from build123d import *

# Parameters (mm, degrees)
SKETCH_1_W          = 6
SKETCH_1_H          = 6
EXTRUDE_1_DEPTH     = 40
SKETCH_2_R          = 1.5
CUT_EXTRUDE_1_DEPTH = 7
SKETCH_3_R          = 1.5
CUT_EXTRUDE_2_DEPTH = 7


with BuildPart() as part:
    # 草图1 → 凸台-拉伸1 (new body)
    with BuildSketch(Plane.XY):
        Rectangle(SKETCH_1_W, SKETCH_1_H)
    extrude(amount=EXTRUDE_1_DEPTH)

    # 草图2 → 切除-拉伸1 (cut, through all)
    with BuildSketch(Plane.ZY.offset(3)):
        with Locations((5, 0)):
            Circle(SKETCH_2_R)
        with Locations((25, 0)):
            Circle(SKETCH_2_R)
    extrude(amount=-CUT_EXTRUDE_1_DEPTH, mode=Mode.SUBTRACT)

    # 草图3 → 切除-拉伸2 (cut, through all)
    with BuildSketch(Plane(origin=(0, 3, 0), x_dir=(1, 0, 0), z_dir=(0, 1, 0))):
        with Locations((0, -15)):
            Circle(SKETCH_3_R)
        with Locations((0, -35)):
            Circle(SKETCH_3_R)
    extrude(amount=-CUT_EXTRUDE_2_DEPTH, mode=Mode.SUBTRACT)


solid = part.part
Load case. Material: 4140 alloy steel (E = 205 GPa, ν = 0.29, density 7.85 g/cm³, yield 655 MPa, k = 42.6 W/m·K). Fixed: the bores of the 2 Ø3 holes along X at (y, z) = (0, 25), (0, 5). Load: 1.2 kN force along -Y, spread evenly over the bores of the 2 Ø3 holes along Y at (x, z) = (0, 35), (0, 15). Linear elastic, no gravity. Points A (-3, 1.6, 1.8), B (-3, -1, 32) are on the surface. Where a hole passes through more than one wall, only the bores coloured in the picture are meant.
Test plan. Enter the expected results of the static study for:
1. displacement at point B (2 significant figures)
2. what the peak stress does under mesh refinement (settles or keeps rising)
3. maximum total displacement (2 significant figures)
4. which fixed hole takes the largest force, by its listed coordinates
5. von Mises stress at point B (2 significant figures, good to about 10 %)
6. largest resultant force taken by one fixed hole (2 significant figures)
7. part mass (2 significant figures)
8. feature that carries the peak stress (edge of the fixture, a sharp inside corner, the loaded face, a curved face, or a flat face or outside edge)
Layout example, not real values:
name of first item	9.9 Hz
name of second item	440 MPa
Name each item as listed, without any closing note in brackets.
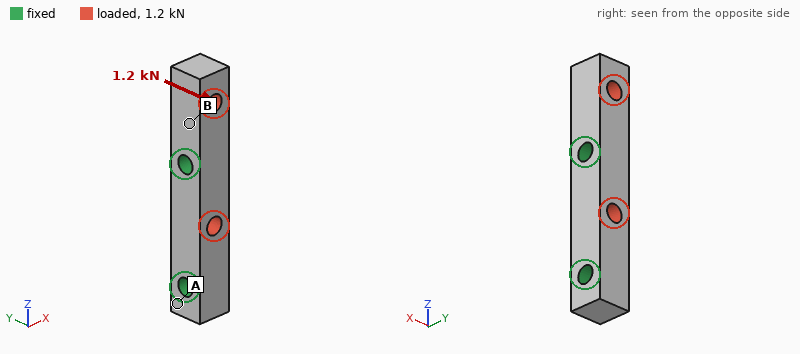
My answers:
displacement at point B	6.7 µm
what the peak stress does under mesh refinement	keeps rising
maximum total displacement	20 µm
which fixed hole takes the largest force, by its listed coordinates	(0, 25)
von Mises stress at point B	45 MPa
largest resultant force taken by one fixed hole	940 N
part mass	10.0 g
feature that carries the peak stress	edge of the fixture
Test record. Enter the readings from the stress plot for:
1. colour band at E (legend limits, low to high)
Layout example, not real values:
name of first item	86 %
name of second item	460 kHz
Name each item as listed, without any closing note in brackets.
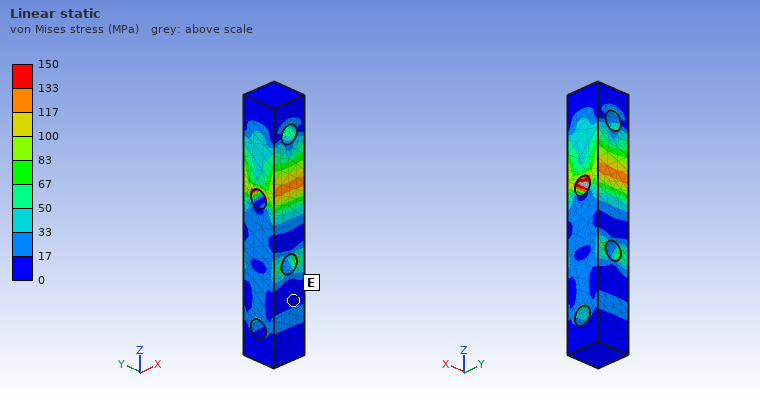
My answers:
colour band at E	0 to 17 MPa
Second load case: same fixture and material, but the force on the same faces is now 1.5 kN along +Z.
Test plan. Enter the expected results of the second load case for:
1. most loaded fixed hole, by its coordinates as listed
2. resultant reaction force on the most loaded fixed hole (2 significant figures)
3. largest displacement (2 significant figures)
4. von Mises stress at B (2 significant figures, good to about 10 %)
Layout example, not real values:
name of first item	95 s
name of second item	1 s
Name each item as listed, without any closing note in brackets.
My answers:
most loaded fixed hole, by its coordinates as listed	(0, 25)
resultant reaction force on the most loaded fixed hole	1.1 kN
largest displacement	1.4 µm
von Mises stress at B	25 MPa
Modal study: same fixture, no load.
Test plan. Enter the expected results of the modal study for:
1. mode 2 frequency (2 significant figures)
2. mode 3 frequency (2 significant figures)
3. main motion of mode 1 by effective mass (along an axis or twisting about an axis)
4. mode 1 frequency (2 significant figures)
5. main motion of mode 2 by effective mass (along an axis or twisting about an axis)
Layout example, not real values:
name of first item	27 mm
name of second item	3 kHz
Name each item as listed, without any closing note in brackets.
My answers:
mode 2 frequency	22 kHz
mode 3 frequency	50 kHz
main motion of mode 1 by effective mass	along Y
mode 1 frequency	20 kHz
main motion of mode 2 by effective mass	along X
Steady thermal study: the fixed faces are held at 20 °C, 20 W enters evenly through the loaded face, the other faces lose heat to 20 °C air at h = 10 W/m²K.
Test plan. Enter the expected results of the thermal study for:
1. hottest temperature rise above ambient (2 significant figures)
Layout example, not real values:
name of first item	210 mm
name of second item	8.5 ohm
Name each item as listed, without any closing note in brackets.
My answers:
hottest temperature rise above ambient	71 K
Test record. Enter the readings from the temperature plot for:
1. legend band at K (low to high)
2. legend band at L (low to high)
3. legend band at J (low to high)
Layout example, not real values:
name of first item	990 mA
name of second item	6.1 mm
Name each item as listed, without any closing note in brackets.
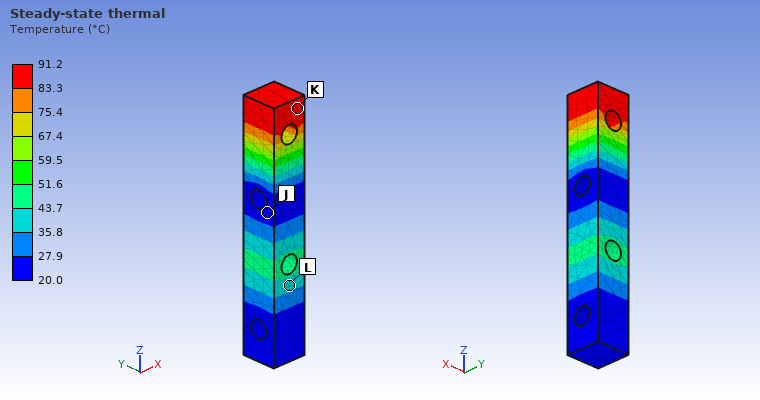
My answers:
legend band at K	83.3 to 91.2 °C
legend band at L	35.8 to 43.7 °C
legend band at J	20.0 to 27.9 °C
